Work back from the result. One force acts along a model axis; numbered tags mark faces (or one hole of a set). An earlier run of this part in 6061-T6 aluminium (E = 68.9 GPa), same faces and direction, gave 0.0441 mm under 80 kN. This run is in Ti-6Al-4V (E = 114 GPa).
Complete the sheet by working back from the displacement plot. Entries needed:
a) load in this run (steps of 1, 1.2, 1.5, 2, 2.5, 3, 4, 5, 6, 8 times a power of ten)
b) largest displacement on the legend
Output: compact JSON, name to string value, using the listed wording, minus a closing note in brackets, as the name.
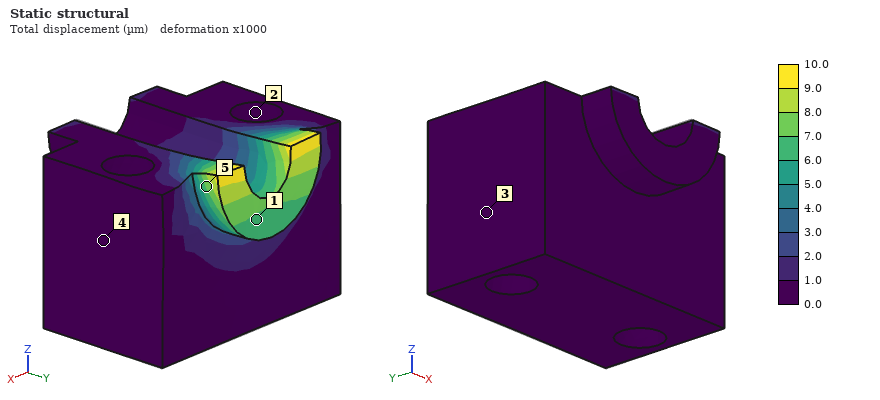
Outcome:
{"load in this run": "30 kN", "largest displacement on the legend": "10.0 µm"}
